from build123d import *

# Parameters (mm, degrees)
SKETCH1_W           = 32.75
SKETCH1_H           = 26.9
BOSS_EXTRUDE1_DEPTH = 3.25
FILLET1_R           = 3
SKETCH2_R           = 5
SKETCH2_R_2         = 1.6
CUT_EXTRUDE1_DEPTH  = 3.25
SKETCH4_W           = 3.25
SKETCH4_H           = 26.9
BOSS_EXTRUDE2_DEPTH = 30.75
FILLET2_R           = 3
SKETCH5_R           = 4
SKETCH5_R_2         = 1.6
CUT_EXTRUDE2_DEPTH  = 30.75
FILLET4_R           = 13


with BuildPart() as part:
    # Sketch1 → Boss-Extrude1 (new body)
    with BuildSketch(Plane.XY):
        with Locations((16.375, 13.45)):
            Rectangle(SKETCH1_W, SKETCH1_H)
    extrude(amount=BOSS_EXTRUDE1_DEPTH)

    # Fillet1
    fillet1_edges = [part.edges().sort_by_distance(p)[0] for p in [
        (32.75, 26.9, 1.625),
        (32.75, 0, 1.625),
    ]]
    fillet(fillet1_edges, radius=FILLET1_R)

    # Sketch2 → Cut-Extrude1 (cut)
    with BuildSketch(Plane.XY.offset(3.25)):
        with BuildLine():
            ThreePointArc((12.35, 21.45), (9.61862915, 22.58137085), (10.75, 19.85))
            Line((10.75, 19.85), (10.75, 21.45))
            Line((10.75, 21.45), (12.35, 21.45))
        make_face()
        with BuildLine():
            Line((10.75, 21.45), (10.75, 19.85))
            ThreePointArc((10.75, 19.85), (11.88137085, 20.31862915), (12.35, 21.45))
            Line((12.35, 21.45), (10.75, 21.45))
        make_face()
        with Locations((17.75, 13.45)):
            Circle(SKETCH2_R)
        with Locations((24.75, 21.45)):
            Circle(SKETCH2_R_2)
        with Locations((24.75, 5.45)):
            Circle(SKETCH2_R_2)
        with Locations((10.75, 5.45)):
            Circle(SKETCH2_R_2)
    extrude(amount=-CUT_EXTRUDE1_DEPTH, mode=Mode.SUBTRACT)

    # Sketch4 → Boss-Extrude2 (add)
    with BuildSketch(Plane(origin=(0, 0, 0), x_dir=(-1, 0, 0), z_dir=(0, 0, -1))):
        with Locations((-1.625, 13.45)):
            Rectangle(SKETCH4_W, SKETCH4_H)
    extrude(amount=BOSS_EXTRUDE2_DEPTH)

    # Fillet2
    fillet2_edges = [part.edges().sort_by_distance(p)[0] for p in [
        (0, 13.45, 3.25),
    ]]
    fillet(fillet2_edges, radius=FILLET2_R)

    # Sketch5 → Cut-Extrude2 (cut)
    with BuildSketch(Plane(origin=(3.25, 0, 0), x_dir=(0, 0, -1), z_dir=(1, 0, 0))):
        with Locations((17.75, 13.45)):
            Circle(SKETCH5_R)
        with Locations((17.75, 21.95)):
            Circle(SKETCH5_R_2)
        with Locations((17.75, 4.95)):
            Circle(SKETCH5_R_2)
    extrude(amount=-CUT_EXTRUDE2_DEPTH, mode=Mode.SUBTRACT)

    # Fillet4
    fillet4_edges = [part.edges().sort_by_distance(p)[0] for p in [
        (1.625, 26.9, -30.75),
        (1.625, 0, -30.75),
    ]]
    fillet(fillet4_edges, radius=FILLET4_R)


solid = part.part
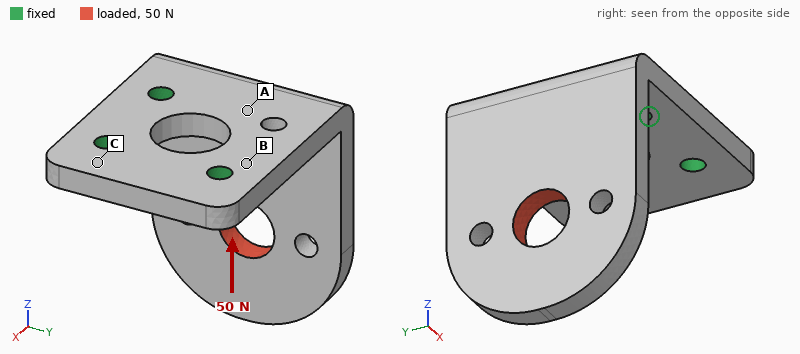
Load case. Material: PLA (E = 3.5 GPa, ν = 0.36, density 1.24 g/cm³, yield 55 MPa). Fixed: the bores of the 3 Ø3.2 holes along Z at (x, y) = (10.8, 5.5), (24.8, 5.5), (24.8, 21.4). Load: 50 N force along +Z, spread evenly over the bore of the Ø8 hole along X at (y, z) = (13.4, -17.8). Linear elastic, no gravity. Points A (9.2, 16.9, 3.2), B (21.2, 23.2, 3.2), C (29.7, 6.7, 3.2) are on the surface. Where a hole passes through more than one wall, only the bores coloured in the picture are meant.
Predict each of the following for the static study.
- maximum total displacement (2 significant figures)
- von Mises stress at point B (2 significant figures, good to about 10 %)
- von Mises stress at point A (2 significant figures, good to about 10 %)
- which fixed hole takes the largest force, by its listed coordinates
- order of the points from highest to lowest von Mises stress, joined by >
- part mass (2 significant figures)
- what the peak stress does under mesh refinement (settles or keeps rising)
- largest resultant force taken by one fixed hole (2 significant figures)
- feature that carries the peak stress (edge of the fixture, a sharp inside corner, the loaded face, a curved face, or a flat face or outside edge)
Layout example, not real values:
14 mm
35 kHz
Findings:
0.57 mm
7.0 MPa
3.6 MPa
(10.8, 5.5)
B > A > C
5.8 g
keeps rising
50 N
edge of the fixture
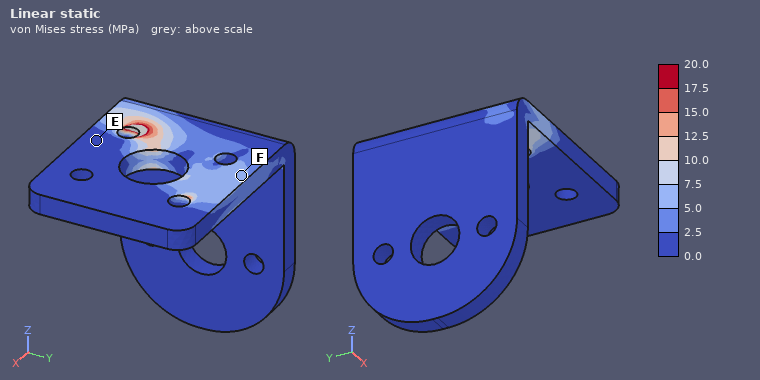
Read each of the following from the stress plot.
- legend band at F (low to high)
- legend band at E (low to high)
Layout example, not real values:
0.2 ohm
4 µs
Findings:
5.0 to 7.5 MPa
0.0 to 2.5 MPa
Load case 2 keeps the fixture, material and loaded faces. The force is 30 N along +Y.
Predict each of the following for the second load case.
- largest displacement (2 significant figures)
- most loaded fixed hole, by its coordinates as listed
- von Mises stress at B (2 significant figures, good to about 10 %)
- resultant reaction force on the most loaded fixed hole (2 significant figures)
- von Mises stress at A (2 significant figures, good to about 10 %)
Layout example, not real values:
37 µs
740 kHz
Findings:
0.52 mm
(10.8, 5.5)
9.2 MPa
33 N
3.7 MPa
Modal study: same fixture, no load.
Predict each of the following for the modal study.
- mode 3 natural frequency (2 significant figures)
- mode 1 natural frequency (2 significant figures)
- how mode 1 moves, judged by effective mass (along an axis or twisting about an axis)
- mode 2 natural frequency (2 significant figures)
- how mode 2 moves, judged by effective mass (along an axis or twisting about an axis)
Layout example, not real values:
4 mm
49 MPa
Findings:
2400 Hz
620 Hz
along X
1000 Hz
along Y
